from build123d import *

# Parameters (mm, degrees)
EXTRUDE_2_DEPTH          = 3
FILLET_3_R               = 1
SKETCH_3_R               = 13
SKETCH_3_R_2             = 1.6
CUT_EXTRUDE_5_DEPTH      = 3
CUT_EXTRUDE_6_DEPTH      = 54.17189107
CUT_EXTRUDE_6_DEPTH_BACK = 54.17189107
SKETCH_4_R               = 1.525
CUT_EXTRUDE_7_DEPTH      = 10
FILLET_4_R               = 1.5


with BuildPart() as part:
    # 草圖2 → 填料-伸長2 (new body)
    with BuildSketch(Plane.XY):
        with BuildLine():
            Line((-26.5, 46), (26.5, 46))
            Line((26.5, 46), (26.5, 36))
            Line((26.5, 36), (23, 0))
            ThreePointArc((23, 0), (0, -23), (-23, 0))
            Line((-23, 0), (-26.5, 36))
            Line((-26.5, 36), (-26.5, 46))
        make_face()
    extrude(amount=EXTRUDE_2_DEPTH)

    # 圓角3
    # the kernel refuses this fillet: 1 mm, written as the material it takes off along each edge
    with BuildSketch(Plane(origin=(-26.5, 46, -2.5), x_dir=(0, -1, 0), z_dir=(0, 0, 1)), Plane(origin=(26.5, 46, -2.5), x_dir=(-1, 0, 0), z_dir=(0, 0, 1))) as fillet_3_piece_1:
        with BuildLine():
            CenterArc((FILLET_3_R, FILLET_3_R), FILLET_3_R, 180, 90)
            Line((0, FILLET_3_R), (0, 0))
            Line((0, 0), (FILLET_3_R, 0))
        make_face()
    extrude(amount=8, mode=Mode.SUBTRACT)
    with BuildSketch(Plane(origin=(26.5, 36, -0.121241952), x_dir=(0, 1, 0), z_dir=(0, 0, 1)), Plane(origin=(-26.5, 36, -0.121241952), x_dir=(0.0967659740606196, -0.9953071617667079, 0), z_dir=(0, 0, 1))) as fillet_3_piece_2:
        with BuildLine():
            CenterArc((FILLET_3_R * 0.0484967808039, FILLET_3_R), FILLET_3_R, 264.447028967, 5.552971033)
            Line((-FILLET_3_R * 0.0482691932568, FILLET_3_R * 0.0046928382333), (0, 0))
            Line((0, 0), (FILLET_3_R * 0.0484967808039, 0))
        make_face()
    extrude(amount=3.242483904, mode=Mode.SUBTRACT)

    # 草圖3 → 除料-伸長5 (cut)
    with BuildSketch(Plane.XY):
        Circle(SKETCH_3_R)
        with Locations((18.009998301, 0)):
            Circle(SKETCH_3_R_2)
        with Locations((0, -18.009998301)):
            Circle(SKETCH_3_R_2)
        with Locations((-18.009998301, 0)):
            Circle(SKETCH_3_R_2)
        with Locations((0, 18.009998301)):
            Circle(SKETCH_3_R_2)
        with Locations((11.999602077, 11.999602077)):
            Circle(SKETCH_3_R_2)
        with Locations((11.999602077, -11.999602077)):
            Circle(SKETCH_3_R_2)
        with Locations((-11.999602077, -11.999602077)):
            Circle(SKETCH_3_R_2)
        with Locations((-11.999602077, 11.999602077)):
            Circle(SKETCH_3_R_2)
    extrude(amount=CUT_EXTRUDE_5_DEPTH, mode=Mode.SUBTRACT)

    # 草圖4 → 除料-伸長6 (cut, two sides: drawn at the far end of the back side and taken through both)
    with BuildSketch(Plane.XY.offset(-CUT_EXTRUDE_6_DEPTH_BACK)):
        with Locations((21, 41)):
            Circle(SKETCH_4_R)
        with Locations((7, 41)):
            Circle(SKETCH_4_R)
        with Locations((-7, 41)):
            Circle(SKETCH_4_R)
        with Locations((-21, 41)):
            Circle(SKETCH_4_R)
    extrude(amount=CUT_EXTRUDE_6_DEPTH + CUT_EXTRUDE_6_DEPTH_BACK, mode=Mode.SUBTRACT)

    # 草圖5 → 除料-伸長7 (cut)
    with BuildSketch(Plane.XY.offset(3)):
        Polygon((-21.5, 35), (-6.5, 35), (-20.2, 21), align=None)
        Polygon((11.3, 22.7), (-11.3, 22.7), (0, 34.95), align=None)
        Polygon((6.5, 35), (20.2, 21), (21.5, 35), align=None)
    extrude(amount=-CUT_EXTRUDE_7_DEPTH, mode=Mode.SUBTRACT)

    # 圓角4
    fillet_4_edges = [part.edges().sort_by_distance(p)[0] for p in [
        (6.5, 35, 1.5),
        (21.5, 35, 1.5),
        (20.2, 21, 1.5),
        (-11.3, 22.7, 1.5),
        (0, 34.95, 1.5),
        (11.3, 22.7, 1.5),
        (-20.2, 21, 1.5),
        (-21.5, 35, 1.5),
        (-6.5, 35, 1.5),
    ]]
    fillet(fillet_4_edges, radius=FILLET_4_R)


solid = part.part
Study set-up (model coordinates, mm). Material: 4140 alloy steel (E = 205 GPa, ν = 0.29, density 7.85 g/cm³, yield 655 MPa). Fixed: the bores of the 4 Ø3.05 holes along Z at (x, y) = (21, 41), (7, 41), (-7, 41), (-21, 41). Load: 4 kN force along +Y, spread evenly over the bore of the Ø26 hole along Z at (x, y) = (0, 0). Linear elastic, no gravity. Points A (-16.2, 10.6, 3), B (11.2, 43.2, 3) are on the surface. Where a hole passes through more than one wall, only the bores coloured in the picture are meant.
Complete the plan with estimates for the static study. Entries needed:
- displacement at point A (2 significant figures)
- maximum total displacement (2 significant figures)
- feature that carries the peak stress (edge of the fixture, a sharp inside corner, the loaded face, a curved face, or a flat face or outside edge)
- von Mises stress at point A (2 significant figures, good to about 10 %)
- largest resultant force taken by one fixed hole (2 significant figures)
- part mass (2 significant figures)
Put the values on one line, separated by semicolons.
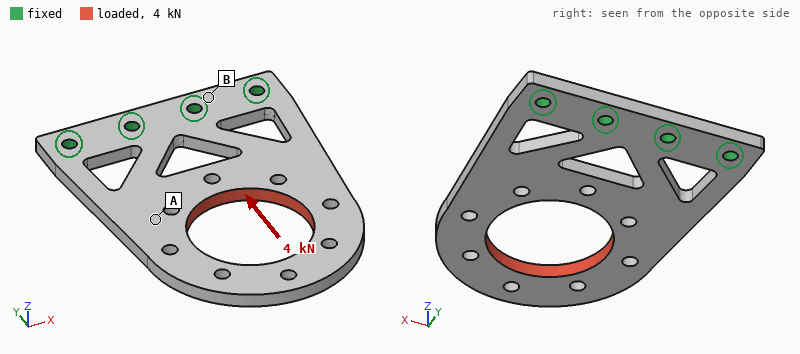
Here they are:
11 µm; 20 µm; a curved face; 40 MPa; 1.1 kN; 51 g
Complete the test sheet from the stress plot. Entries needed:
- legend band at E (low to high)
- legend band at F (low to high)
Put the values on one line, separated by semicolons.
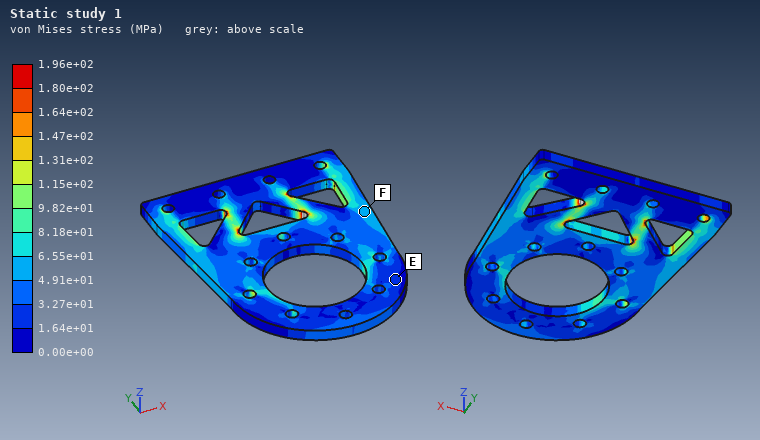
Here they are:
1.64e+01 to 3.27e+01 MPa; 4.91e+01 to 6.55e+01 MPa
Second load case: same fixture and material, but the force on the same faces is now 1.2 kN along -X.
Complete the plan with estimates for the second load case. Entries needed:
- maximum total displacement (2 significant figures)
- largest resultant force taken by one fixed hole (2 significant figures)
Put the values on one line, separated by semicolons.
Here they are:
38 µm; 1.1 kN
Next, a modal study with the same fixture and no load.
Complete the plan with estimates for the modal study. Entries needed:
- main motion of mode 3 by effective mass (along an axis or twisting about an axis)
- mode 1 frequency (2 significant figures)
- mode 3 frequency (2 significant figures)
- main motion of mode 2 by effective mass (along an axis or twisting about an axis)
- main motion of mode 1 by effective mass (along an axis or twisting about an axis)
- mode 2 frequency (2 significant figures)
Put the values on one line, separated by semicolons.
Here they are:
along Z; 620 Hz; 3400 Hz; twisting about Y; along Z; 2000 Hz
